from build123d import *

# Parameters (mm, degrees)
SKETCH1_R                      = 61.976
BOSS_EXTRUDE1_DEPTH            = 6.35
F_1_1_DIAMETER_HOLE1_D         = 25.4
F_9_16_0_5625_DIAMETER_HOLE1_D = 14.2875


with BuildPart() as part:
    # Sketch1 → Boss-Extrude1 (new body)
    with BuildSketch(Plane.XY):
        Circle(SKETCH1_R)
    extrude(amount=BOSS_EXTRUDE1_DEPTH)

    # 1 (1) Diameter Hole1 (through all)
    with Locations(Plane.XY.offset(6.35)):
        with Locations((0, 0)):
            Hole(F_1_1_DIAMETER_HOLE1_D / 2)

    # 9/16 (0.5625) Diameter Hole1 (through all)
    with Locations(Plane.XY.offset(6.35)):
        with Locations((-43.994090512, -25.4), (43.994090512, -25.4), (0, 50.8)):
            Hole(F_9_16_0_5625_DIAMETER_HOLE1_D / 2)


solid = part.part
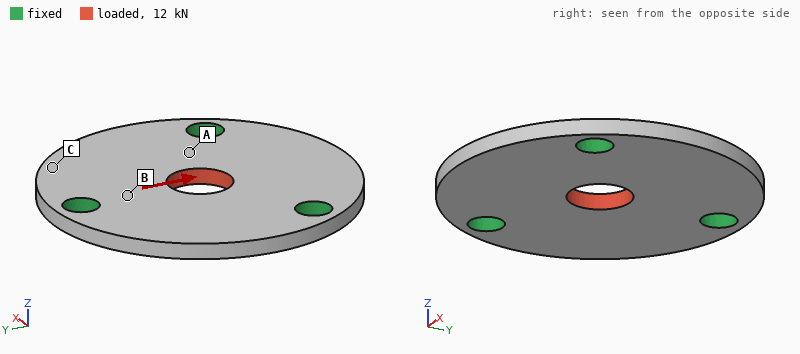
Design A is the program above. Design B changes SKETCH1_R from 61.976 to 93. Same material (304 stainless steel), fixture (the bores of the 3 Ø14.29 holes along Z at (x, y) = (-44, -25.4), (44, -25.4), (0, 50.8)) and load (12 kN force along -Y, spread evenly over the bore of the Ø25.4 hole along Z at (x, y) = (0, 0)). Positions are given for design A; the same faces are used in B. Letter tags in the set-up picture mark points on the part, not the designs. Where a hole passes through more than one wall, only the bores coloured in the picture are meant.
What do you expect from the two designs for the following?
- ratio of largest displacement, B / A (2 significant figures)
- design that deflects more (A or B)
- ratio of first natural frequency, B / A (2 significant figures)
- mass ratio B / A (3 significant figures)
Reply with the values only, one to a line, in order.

0.82
A
0.41
2.36
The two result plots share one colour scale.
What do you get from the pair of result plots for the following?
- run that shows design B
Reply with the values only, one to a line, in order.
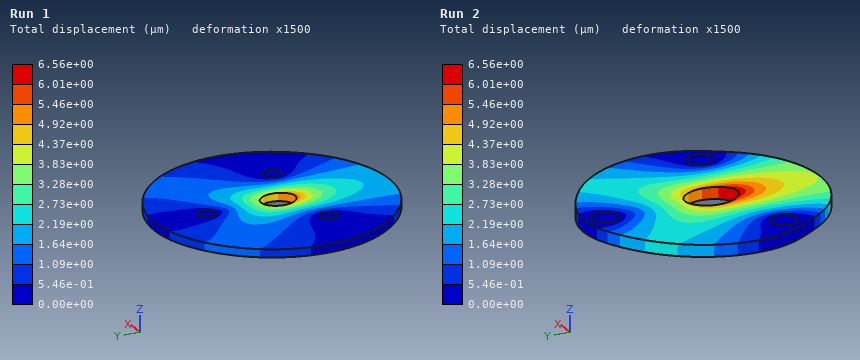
Run 1
